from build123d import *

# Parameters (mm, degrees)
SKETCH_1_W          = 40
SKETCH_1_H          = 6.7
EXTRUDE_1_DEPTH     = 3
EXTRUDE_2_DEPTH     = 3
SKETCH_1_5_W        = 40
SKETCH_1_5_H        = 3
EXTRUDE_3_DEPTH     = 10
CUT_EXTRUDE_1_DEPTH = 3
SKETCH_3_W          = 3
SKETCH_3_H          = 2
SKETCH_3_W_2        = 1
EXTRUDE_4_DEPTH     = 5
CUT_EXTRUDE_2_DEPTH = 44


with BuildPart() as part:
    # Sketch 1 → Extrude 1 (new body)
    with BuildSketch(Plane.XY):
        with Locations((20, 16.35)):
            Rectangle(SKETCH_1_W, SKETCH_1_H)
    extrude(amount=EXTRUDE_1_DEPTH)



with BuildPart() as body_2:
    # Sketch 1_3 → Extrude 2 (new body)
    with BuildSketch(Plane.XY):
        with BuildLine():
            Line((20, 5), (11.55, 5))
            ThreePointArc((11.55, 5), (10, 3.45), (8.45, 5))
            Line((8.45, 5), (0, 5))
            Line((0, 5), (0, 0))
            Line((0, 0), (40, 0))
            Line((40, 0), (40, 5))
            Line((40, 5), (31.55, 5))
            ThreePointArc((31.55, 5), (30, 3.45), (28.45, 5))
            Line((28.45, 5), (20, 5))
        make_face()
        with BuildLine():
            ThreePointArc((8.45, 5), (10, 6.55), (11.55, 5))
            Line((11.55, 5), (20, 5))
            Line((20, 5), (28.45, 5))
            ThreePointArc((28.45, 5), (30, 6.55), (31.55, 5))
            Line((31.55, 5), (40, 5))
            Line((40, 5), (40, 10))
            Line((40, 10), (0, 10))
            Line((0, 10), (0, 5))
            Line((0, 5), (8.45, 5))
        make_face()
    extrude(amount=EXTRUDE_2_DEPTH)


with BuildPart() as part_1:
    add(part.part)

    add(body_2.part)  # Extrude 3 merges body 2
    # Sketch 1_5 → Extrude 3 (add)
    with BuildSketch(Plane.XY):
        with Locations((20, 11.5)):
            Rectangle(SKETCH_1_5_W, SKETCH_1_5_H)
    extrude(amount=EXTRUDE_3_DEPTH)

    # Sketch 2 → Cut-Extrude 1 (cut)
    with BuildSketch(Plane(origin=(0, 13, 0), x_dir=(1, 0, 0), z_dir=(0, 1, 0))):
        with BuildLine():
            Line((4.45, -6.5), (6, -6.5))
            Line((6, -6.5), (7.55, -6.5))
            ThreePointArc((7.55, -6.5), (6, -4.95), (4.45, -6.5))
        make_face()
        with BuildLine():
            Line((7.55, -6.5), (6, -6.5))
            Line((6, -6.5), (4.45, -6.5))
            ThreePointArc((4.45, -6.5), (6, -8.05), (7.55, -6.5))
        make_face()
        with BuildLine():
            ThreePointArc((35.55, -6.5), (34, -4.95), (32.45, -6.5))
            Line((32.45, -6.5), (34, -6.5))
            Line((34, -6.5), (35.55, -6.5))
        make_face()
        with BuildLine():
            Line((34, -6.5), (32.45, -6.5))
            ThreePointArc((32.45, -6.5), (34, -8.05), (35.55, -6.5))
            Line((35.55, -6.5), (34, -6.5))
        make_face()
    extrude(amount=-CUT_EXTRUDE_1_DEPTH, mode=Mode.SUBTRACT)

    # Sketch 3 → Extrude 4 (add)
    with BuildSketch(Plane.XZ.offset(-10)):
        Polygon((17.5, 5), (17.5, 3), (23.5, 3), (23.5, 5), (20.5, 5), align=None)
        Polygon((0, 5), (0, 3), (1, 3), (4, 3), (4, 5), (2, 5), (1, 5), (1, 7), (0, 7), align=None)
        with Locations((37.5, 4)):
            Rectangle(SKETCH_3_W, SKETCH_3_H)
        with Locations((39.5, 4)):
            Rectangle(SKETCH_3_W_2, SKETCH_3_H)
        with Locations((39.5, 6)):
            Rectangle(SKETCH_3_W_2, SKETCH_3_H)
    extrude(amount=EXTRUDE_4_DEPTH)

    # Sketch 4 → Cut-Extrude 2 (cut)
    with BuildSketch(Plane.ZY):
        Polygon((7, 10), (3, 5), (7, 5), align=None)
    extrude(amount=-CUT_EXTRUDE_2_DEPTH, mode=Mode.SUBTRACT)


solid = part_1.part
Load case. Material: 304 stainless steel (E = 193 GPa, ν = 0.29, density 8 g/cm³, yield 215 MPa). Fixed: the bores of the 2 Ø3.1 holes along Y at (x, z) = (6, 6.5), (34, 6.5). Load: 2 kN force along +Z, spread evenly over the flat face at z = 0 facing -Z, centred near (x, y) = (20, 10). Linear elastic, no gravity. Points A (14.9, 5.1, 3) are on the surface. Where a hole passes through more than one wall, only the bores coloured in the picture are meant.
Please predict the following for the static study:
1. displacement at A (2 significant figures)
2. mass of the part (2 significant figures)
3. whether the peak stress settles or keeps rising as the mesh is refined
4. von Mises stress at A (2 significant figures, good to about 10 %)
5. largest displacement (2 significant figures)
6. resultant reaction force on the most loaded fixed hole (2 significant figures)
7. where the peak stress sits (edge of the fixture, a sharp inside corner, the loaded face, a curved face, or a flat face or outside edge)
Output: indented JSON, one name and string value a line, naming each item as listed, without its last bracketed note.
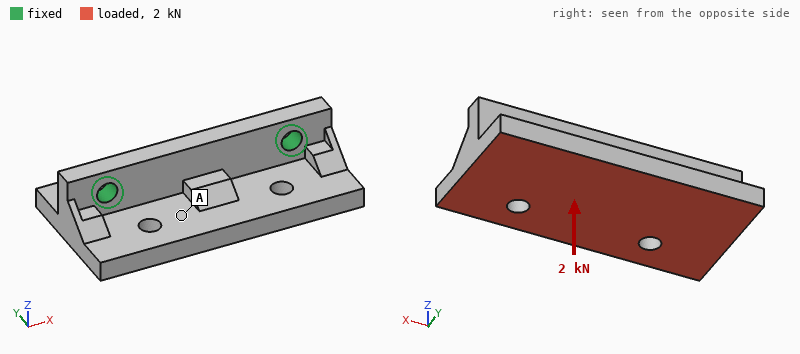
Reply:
{
  "displacement at A": "11 µm",
  "mass of the part": "26 g",
  "whether the peak stress settles or keeps rising as the mesh is refined": "keeps rising",
  "von Mises stress at A": "17 MPa",
  "largest displacement": "21 µm",
  "resultant reaction force on the most loaded fixed hole": "1.1 kN",
  "where the peak stress sits": "edge of the fixture"
}
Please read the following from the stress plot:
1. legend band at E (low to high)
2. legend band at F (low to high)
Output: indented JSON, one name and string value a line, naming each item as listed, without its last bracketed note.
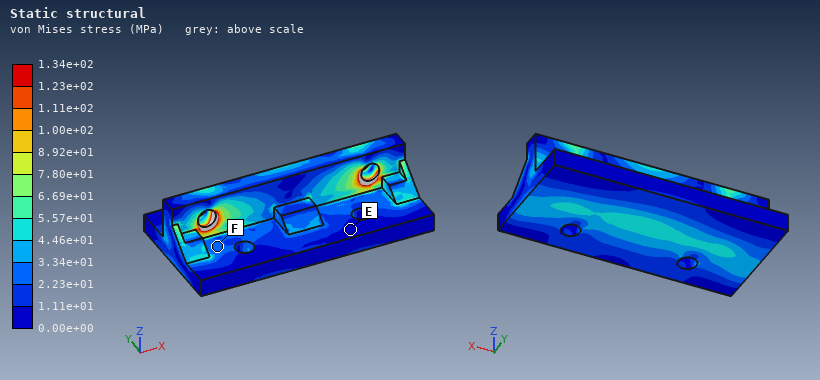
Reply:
{
  "legend band at E": "0.00e+00 to 1.11e+01 MPa",
  "legend band at F": "2.23e+01 to 3.34e+01 MPa"
}
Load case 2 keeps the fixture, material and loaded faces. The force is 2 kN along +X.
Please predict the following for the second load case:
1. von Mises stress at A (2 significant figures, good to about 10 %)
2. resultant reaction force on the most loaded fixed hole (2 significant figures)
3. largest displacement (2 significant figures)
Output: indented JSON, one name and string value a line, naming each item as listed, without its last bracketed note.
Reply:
{
  "von Mises stress at A": "11 MPa",
  "resultant reaction force on the most loaded fixed hole": "1.1 kN",
  "largest displacement": "3.8 µm"
}
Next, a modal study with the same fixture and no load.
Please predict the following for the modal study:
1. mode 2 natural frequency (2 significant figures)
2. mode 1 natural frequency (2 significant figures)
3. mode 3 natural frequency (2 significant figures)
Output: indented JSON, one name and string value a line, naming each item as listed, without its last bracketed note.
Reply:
{
  "mode 2 natural frequency": "15 kHz",
  "mode 1 natural frequency": "9500 Hz",
  "mode 3 natural frequency": "21 kHz"
}
